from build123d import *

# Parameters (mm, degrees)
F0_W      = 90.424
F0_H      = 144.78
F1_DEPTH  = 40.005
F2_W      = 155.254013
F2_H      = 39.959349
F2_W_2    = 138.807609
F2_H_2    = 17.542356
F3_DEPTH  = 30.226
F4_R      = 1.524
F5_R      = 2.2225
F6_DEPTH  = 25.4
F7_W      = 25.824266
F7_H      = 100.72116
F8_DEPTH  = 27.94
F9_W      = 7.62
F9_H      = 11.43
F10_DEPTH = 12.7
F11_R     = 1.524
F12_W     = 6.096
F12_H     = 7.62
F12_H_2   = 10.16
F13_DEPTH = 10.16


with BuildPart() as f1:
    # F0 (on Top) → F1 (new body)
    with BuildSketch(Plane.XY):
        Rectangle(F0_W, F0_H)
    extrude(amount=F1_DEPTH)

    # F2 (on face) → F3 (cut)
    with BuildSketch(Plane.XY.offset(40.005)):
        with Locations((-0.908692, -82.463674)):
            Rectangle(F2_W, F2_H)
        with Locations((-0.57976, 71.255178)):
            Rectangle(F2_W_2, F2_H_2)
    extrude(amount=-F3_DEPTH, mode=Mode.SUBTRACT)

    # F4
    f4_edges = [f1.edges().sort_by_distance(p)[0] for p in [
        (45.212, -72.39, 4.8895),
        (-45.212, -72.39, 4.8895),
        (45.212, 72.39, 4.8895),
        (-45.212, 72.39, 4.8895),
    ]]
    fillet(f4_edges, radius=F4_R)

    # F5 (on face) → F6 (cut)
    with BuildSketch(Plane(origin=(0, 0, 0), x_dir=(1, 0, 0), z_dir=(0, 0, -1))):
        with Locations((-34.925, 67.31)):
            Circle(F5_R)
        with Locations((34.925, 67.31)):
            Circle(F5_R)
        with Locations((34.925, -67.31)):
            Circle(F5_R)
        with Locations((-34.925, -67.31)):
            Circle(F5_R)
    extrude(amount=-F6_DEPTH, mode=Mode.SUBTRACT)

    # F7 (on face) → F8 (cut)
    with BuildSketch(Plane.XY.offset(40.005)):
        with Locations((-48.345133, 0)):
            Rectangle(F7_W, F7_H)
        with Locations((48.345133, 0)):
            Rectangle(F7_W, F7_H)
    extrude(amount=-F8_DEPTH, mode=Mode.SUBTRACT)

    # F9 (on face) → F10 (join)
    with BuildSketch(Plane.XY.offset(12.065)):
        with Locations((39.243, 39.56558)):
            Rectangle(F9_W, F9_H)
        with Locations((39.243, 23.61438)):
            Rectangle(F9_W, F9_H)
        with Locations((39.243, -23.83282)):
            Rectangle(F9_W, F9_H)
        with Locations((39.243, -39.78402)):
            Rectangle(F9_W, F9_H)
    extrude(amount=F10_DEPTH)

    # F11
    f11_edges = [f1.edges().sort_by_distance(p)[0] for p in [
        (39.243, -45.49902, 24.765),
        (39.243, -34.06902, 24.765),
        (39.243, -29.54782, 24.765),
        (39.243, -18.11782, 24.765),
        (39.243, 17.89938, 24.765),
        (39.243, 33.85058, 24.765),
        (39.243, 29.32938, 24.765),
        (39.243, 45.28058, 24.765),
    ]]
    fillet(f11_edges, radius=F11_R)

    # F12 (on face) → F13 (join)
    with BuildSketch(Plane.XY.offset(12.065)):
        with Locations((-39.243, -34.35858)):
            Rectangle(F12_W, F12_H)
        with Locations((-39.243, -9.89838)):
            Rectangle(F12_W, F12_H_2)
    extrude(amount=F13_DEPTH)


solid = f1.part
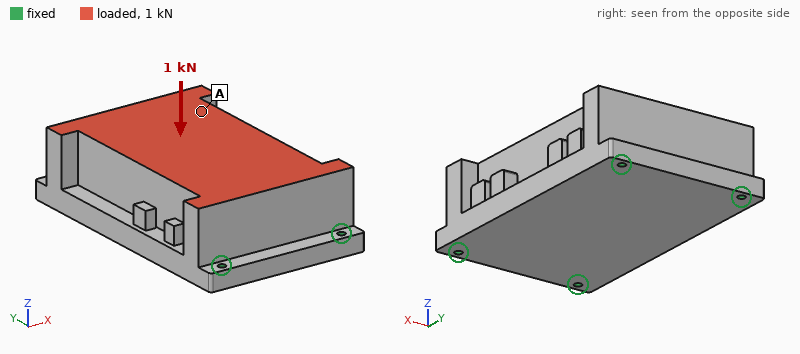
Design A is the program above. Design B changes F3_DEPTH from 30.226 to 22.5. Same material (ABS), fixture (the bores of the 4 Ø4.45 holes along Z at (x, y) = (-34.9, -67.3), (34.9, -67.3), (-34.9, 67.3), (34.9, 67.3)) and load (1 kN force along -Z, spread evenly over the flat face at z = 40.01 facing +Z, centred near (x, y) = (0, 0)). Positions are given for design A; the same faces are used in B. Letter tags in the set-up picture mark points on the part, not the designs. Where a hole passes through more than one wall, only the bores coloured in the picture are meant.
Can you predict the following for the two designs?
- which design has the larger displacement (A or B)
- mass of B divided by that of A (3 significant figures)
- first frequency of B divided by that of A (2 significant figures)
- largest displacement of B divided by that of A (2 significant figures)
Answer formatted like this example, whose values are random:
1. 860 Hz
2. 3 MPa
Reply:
1. A
2. 1.03
3. 1.2
4. 0.77
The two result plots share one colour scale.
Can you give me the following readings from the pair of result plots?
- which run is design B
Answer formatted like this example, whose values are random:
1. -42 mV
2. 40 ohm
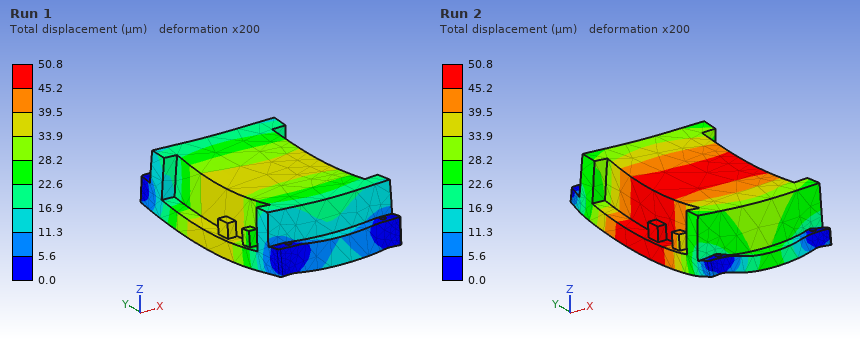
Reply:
1. Run 1
